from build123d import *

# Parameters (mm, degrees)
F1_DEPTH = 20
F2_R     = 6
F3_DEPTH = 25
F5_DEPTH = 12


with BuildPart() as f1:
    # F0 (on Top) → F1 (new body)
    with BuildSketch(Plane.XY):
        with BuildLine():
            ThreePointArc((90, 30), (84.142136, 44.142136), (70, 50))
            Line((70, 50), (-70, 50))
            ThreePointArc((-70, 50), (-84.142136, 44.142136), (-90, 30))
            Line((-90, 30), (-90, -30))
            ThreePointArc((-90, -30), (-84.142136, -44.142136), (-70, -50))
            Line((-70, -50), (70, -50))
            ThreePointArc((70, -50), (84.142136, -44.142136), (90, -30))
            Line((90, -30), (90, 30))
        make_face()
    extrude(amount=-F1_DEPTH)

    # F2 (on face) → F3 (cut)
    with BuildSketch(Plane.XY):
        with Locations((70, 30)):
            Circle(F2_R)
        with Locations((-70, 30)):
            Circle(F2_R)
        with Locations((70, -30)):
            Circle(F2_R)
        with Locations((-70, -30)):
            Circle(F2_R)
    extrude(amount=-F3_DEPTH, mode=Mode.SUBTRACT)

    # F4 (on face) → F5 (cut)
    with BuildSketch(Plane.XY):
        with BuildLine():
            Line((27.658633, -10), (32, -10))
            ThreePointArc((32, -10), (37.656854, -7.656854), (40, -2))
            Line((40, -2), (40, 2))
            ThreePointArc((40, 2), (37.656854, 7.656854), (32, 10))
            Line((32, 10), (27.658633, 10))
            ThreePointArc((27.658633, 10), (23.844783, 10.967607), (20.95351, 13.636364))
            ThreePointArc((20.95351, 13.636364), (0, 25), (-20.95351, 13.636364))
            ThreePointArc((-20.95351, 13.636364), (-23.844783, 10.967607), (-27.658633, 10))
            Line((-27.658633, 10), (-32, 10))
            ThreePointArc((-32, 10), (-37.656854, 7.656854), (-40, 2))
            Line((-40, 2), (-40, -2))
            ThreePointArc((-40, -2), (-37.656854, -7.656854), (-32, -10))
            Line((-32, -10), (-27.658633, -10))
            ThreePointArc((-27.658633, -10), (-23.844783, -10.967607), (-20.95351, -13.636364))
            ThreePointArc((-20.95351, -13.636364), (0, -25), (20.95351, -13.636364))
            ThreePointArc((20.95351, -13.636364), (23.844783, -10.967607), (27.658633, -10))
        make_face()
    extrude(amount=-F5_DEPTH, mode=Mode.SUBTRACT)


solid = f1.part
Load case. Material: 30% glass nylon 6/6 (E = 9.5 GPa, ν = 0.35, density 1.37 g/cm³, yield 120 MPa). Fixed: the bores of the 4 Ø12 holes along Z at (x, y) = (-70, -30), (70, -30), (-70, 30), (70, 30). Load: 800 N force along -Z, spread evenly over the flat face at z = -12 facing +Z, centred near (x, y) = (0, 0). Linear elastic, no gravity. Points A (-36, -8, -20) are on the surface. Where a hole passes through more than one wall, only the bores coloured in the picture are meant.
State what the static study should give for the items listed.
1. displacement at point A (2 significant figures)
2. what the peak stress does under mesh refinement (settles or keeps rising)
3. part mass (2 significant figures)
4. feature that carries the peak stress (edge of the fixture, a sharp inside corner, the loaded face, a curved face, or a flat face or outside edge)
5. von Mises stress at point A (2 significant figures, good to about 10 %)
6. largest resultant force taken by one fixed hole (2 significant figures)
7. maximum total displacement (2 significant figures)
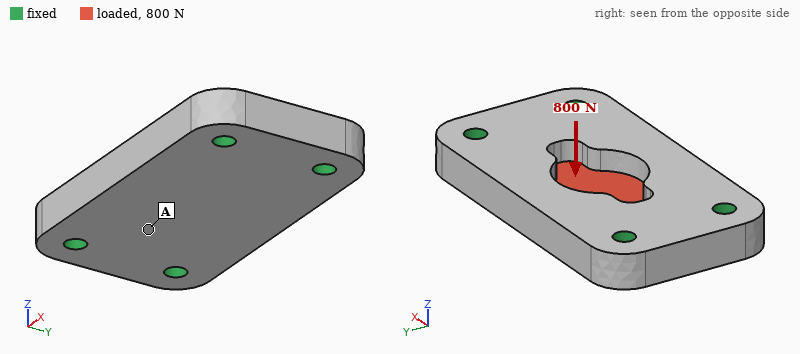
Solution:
15 µm
keeps rising
430 g
edge of the fixture
0.64 MPa
220 N
37 µm
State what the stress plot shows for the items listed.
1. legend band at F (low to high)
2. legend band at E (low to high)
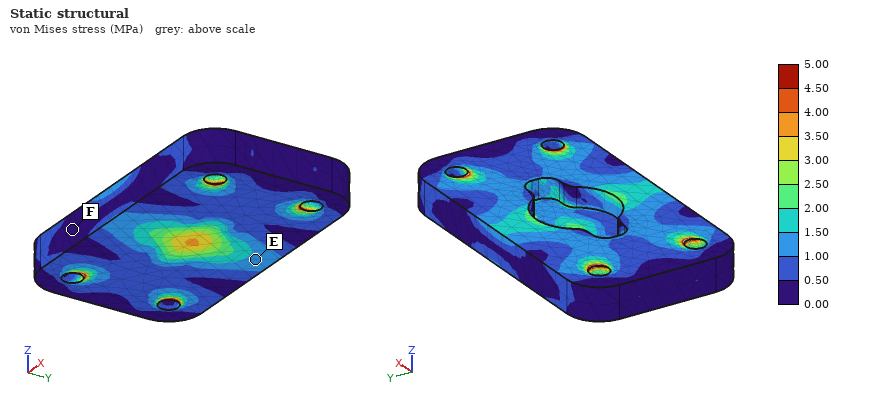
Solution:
0.00 to 0.50 MPa
1.00 to 1.50 MPa
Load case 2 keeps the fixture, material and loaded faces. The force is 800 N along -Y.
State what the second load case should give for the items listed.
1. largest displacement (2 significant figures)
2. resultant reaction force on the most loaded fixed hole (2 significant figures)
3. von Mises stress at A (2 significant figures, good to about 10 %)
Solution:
7.4 µm
250 N
0.56 MPa
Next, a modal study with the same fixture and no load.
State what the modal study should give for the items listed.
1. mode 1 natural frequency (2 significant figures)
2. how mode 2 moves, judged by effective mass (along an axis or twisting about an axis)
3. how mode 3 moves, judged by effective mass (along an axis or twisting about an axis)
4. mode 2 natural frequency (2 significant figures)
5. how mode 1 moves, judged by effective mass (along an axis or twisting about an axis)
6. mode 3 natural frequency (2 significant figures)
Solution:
2500 Hz
twisting about X
along Y
3000 Hz
along Z
5000 Hz
